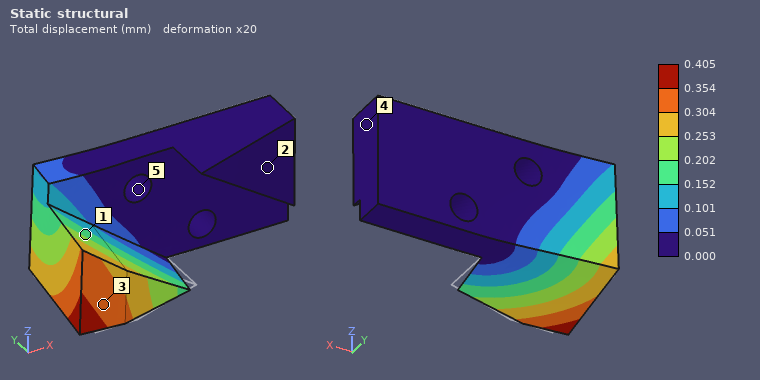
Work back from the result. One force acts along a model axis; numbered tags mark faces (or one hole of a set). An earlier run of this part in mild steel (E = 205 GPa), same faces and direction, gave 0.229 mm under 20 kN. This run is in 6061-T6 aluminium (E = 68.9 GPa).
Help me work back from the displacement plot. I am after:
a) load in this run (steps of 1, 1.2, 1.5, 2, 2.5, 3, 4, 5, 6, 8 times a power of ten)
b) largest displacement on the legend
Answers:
12 kN
0.405 mm
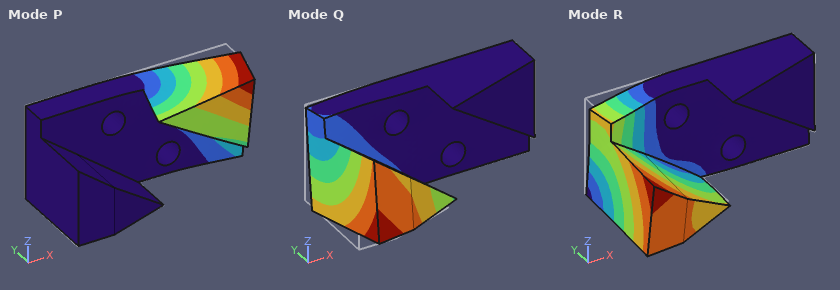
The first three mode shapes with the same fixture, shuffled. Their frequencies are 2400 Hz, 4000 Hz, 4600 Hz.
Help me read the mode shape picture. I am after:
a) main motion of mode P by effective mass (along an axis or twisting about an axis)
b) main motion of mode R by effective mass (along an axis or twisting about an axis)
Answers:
along Y
along Z
